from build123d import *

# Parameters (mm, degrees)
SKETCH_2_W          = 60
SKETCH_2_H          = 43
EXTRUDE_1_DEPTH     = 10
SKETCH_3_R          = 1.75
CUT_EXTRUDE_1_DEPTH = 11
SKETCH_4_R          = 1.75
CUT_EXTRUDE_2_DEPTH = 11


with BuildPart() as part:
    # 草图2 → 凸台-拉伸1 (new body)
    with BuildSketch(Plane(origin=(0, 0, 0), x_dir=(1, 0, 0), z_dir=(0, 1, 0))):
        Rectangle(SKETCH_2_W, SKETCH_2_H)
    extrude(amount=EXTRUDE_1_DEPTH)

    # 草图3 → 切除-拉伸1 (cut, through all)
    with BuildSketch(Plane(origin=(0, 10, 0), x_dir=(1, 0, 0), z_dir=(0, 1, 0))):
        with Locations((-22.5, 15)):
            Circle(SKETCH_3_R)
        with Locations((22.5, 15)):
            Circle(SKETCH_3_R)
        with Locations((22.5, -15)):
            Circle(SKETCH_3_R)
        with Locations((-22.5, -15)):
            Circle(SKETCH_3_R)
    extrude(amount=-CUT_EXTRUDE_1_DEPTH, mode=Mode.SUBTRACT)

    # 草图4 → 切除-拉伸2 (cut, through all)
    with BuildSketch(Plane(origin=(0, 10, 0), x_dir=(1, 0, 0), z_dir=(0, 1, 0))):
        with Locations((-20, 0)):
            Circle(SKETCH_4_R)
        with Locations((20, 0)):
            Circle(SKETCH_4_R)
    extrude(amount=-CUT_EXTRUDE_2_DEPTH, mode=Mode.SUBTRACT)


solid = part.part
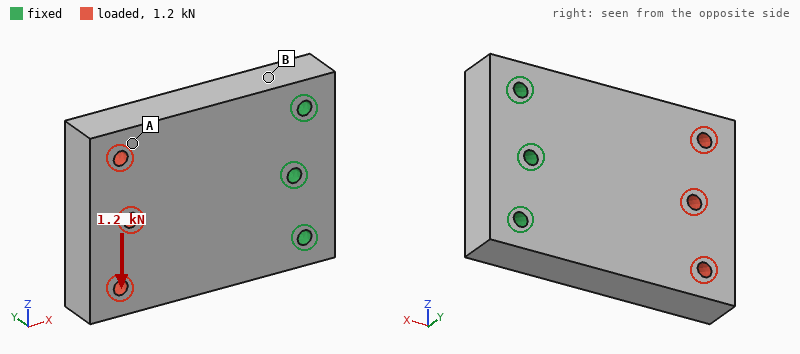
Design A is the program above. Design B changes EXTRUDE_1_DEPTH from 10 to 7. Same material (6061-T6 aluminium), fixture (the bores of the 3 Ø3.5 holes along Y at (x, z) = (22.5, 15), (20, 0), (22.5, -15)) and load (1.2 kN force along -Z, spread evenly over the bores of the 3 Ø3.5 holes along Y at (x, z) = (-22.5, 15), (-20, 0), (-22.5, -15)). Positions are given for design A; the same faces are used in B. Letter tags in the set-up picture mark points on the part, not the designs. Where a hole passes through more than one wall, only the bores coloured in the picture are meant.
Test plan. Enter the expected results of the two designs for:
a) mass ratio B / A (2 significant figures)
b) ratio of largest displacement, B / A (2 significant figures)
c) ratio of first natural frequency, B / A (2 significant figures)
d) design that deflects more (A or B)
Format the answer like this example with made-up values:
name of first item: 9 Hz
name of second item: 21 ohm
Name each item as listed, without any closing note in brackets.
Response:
mass ratio B / A: 0.70
ratio of largest displacement, B / A: 1.4
ratio of first natural frequency, B / A: 0.72
design that deflects more: B
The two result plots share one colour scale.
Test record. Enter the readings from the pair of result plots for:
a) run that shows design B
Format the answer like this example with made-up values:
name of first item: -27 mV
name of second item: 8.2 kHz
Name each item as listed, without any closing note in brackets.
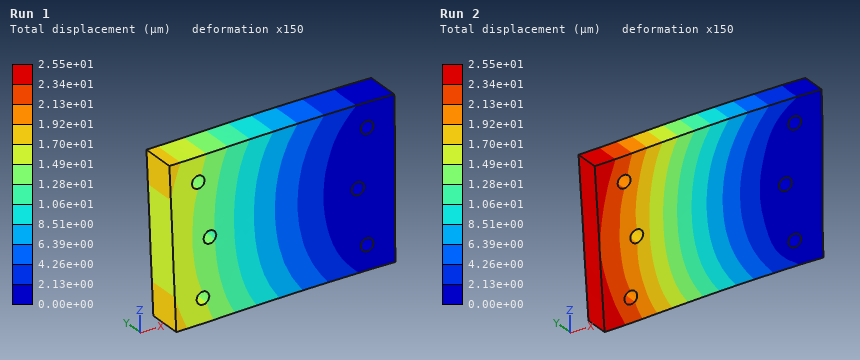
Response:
run that shows design B: Run 2
